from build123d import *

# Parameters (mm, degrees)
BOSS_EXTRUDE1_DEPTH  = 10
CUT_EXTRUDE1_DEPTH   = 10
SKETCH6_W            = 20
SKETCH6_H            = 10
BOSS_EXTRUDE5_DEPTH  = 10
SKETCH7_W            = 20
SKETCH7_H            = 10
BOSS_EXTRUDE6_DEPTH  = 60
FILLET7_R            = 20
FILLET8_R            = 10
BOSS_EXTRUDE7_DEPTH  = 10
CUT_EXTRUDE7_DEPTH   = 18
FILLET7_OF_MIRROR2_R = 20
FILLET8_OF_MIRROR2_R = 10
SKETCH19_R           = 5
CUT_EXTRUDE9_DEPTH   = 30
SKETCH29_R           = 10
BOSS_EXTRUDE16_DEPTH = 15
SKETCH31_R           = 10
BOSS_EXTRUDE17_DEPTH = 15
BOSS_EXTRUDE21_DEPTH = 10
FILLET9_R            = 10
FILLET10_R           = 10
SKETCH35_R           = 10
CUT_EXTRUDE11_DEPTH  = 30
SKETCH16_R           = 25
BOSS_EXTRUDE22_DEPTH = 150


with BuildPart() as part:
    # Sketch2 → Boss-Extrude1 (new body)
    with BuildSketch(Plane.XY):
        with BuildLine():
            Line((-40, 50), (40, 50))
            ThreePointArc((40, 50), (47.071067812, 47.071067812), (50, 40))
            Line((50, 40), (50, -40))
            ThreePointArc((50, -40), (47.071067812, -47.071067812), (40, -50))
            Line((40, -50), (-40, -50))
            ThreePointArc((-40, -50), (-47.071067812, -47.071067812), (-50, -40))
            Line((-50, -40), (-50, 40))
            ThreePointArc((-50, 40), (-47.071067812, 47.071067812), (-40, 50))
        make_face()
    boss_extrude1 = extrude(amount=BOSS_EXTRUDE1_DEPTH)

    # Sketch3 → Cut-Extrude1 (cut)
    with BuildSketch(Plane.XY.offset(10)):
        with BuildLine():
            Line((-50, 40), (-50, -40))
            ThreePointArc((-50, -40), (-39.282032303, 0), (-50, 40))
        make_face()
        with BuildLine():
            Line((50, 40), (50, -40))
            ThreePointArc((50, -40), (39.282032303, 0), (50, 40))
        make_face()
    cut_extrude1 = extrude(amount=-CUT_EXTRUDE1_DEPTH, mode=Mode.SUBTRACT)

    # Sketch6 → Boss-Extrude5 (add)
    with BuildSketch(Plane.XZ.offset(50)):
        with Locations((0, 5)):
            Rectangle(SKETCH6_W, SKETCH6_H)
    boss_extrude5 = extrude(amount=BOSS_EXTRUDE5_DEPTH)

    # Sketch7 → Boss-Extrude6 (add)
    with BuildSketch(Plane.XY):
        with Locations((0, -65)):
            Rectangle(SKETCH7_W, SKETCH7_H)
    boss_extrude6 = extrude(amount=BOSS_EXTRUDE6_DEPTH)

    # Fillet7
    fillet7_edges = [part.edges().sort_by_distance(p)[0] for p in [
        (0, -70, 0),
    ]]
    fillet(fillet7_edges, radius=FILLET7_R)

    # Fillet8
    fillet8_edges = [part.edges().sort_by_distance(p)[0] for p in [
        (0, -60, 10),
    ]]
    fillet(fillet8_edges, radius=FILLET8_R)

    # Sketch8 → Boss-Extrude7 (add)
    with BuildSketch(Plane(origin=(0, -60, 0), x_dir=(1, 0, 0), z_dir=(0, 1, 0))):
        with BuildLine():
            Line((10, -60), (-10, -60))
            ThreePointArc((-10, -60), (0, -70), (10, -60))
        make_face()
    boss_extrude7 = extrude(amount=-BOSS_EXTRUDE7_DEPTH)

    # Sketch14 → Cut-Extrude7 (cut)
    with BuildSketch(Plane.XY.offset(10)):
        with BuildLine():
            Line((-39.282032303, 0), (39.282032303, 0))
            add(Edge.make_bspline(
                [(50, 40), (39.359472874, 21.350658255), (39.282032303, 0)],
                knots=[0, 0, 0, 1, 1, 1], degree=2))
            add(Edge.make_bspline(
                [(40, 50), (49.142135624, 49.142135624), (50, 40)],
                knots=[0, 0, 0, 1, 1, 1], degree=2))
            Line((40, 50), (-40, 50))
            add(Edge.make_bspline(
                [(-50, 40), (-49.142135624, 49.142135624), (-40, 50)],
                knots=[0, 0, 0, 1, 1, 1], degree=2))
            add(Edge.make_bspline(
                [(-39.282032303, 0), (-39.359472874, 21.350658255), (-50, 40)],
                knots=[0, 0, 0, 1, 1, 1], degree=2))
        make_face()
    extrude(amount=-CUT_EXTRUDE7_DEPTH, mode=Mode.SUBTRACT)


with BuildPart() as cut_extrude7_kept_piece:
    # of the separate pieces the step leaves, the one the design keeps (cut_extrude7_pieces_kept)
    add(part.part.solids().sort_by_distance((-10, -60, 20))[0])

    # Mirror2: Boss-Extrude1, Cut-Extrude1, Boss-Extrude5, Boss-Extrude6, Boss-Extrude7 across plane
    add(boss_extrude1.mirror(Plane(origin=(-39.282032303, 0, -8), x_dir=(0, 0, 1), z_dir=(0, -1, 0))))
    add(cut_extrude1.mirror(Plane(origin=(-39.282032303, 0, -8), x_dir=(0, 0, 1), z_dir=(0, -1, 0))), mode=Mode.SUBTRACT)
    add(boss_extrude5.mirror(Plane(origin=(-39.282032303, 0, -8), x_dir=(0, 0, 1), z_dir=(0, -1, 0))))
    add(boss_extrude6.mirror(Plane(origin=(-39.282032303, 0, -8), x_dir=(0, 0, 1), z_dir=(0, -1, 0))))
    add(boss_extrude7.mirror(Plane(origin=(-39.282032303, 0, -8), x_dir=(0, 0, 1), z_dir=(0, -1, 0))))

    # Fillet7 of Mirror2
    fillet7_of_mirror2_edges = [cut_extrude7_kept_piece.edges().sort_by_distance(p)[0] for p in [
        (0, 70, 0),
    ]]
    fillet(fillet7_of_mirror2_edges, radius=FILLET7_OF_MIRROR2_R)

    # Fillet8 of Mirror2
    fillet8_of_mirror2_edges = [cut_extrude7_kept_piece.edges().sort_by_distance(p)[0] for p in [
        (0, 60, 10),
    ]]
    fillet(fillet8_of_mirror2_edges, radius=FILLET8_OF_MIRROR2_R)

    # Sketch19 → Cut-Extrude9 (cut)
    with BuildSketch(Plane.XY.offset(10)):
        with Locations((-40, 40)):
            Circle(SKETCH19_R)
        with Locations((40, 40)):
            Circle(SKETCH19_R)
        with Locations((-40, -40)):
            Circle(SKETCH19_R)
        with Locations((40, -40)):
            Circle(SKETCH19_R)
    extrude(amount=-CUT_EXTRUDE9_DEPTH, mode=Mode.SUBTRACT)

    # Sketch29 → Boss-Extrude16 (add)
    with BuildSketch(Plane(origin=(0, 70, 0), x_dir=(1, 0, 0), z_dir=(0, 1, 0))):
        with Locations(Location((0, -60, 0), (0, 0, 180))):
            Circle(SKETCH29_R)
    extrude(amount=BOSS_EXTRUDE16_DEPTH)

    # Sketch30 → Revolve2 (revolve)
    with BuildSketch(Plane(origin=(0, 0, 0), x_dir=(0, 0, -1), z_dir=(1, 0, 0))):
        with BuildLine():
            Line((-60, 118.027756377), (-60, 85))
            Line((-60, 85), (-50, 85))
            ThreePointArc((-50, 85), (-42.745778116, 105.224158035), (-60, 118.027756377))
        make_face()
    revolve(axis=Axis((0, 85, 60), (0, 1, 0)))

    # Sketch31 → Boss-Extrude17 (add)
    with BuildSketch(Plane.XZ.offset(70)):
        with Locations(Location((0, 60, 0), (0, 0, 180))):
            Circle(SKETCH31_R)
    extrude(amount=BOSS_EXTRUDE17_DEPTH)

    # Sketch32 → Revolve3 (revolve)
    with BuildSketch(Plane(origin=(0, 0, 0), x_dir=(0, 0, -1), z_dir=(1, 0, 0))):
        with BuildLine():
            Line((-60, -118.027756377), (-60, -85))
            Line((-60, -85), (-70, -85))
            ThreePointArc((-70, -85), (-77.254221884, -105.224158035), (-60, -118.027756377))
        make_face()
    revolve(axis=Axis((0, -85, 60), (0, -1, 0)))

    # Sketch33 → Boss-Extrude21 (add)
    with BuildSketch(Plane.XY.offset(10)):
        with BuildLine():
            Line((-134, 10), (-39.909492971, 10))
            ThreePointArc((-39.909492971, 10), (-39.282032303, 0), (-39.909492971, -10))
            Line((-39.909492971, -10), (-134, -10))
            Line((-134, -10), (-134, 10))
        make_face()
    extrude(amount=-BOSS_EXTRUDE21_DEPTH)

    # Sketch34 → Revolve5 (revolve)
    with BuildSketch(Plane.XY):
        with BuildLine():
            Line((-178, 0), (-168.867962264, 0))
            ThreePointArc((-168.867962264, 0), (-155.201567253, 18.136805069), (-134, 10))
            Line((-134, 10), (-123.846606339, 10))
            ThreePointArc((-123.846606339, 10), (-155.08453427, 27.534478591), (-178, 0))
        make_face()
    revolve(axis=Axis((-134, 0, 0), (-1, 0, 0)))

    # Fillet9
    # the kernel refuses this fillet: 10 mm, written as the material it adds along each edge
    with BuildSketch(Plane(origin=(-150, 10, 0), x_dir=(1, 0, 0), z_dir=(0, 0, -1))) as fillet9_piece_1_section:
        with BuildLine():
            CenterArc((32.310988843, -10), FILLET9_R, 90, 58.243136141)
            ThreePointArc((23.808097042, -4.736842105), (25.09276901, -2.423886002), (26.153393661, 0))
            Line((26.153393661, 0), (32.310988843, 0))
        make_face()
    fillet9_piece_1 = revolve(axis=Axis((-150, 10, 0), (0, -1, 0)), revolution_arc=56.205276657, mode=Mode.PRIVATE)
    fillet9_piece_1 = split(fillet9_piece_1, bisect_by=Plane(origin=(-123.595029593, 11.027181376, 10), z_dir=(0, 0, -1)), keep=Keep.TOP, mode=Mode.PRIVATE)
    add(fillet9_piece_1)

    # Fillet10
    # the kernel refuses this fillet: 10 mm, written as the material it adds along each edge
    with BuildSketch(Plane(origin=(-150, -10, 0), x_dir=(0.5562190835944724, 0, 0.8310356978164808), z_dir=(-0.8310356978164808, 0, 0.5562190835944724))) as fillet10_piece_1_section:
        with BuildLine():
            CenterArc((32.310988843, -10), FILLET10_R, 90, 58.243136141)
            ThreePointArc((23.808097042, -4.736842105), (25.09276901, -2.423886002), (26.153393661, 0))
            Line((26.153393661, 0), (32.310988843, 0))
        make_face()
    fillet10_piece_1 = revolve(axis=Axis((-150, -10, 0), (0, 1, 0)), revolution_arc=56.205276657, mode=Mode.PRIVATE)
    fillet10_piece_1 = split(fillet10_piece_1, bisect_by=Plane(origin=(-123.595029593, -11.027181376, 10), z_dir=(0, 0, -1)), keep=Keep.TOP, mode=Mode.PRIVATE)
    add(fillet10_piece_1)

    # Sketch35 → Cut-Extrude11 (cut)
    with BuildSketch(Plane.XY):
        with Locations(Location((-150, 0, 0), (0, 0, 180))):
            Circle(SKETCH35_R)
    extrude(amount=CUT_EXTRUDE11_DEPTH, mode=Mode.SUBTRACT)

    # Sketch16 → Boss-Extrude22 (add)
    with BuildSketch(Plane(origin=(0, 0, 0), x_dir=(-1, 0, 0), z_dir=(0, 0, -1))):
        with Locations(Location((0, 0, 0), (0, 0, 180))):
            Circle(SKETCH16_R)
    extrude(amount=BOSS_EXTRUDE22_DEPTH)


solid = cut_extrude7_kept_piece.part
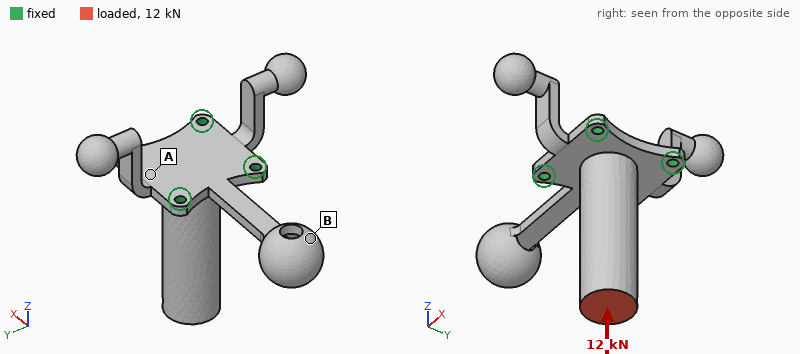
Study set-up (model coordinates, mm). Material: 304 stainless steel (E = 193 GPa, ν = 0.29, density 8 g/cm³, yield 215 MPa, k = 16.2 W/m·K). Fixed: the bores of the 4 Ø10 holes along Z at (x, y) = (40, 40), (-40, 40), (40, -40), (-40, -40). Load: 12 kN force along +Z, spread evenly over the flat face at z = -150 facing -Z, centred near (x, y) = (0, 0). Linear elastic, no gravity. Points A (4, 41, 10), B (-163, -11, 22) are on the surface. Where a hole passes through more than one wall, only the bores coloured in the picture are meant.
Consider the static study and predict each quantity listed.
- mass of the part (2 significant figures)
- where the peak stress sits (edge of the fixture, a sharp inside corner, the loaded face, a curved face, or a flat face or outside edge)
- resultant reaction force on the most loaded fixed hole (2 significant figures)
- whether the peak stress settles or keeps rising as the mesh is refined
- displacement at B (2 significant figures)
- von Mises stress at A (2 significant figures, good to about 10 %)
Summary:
4.3 kg
edge of the fixture
3.1 kN
keeps rising
25 µm
26 MPa
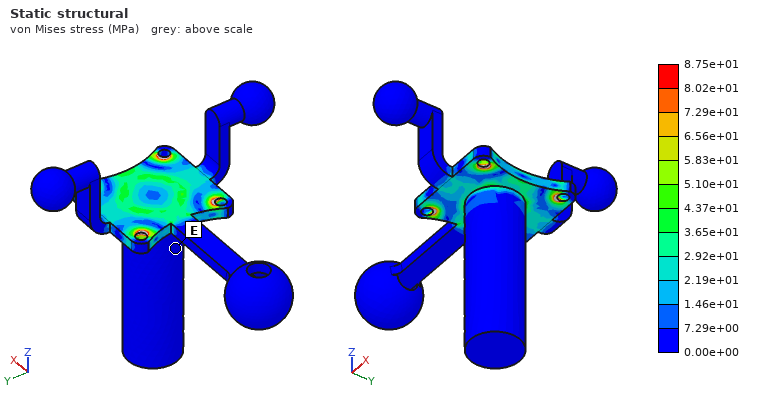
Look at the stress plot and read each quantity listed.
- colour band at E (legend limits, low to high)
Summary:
0.00e+00 to 7.29e+00 MPa
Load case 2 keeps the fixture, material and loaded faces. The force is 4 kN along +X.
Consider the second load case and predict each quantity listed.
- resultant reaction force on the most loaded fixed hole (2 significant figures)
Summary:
4.9 kN
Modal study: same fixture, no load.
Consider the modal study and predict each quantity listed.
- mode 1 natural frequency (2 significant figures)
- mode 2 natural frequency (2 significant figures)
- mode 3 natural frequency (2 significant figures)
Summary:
160 Hz
330 Hz
370 Hz
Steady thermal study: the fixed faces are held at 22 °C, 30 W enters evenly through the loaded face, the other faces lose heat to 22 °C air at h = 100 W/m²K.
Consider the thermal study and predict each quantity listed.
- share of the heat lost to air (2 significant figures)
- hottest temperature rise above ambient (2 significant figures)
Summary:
98 %
45 K
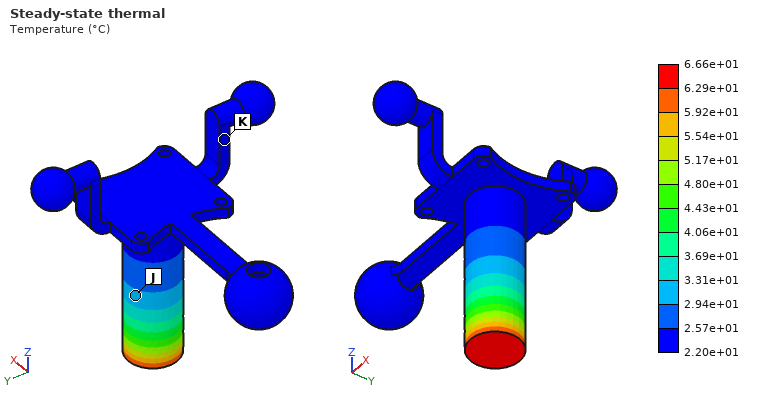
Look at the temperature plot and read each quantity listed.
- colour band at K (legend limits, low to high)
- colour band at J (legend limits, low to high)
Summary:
2.20e+01 to 2.57e+01 °C
2.94e+01 to 3.31e+01 °C
